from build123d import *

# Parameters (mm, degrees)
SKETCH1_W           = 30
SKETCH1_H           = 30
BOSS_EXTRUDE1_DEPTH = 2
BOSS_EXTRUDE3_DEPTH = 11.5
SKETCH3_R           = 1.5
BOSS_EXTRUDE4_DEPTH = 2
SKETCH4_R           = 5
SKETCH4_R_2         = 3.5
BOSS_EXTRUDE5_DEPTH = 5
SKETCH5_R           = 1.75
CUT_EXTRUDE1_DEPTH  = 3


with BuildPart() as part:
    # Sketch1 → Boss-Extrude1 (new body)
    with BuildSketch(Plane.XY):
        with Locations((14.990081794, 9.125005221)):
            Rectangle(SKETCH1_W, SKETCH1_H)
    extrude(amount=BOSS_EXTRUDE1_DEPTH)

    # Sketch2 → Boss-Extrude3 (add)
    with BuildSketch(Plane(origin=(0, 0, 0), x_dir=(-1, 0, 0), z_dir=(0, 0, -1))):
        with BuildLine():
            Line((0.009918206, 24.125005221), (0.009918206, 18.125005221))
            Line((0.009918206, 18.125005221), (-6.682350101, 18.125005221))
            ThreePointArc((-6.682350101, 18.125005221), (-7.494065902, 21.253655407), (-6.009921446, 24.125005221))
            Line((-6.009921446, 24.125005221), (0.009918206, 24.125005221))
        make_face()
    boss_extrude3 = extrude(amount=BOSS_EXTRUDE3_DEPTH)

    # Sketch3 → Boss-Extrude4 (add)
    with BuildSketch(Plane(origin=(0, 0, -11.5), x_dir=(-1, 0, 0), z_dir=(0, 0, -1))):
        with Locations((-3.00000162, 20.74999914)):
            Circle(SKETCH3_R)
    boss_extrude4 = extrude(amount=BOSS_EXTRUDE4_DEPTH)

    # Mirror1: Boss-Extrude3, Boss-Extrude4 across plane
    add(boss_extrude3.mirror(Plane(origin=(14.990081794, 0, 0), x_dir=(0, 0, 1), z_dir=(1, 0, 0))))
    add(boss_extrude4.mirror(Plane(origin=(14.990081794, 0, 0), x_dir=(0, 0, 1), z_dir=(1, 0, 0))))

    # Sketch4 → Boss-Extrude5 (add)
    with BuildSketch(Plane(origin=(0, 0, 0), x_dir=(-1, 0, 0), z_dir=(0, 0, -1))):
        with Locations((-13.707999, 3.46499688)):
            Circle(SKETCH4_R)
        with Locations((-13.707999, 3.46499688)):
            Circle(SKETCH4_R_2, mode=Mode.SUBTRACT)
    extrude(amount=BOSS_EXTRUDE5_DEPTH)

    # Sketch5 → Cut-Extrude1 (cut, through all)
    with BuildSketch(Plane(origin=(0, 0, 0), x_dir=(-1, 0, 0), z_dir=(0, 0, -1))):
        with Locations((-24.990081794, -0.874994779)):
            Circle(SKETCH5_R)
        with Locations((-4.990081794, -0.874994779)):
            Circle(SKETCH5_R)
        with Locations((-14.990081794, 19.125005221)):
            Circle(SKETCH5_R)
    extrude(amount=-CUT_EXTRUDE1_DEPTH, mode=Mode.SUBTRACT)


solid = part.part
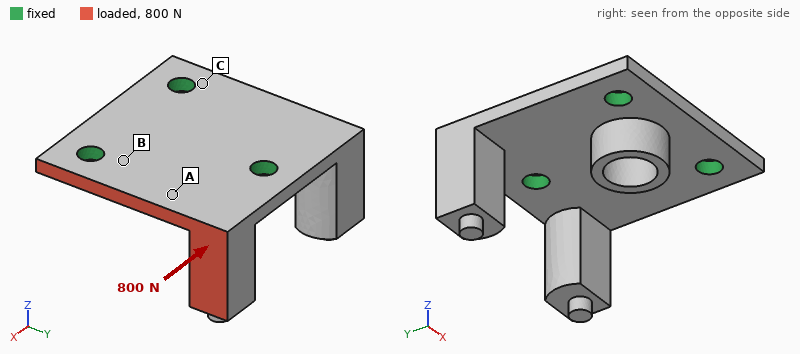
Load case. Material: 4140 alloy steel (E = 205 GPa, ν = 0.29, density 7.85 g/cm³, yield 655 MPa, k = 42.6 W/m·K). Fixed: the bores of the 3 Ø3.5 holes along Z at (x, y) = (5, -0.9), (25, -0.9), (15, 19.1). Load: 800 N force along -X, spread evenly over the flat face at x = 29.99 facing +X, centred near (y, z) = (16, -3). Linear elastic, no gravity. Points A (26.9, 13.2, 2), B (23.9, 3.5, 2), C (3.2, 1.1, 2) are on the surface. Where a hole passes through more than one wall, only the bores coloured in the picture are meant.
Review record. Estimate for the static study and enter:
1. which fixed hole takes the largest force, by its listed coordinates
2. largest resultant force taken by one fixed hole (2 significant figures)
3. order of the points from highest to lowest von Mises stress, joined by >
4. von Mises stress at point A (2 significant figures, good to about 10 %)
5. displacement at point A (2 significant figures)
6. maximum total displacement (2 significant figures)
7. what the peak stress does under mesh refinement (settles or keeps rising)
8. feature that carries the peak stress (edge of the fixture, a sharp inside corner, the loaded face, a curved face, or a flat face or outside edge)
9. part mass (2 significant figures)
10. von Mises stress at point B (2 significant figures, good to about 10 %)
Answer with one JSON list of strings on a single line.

["(15, 19.1)", "590 N", "A > B > C", "180 MPa", "0.037 mm", "0.16 mm", "keeps rising", "edge of the fixture", "23 g", "98 MPa"]
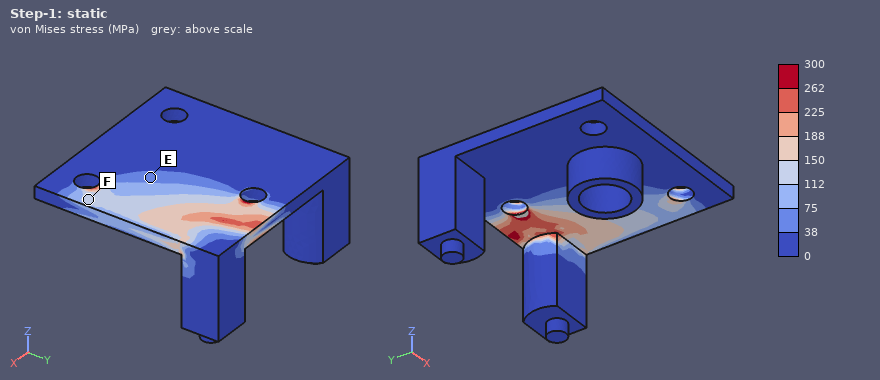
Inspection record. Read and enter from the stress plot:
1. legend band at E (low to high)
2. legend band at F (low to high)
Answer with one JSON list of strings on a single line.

["38 to 75 MPa", "112 to 150 MPa"]
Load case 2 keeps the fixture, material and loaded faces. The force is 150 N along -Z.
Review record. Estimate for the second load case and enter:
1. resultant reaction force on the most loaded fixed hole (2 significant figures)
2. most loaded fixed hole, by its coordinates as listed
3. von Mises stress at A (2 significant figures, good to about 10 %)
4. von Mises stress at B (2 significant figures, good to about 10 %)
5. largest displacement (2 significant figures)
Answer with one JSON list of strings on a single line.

["97 N", "(15, 19.1)", "60 MPa", "49 MPa", "62 µm"]
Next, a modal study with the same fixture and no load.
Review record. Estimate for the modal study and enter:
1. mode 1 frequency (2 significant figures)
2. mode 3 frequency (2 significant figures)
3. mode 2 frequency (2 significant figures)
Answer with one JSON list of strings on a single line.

["3800 Hz", "7000 Hz", "3900 Hz"]
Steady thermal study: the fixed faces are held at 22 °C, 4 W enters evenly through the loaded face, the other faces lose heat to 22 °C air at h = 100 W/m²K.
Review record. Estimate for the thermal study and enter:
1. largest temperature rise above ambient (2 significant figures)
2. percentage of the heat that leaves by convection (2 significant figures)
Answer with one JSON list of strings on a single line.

["24 K", "30 %"]
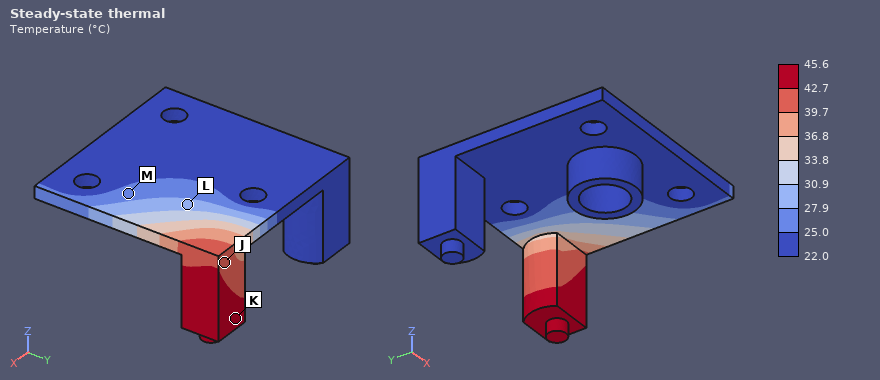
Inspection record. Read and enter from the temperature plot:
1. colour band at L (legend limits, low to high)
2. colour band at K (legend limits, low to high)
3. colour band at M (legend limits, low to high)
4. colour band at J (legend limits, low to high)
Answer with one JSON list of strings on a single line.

["27.9 to 30.9 °C", "42.7 to 45.6 °C", "25.0 to 27.9 °C", "39.7 to 42.7 °C"]
